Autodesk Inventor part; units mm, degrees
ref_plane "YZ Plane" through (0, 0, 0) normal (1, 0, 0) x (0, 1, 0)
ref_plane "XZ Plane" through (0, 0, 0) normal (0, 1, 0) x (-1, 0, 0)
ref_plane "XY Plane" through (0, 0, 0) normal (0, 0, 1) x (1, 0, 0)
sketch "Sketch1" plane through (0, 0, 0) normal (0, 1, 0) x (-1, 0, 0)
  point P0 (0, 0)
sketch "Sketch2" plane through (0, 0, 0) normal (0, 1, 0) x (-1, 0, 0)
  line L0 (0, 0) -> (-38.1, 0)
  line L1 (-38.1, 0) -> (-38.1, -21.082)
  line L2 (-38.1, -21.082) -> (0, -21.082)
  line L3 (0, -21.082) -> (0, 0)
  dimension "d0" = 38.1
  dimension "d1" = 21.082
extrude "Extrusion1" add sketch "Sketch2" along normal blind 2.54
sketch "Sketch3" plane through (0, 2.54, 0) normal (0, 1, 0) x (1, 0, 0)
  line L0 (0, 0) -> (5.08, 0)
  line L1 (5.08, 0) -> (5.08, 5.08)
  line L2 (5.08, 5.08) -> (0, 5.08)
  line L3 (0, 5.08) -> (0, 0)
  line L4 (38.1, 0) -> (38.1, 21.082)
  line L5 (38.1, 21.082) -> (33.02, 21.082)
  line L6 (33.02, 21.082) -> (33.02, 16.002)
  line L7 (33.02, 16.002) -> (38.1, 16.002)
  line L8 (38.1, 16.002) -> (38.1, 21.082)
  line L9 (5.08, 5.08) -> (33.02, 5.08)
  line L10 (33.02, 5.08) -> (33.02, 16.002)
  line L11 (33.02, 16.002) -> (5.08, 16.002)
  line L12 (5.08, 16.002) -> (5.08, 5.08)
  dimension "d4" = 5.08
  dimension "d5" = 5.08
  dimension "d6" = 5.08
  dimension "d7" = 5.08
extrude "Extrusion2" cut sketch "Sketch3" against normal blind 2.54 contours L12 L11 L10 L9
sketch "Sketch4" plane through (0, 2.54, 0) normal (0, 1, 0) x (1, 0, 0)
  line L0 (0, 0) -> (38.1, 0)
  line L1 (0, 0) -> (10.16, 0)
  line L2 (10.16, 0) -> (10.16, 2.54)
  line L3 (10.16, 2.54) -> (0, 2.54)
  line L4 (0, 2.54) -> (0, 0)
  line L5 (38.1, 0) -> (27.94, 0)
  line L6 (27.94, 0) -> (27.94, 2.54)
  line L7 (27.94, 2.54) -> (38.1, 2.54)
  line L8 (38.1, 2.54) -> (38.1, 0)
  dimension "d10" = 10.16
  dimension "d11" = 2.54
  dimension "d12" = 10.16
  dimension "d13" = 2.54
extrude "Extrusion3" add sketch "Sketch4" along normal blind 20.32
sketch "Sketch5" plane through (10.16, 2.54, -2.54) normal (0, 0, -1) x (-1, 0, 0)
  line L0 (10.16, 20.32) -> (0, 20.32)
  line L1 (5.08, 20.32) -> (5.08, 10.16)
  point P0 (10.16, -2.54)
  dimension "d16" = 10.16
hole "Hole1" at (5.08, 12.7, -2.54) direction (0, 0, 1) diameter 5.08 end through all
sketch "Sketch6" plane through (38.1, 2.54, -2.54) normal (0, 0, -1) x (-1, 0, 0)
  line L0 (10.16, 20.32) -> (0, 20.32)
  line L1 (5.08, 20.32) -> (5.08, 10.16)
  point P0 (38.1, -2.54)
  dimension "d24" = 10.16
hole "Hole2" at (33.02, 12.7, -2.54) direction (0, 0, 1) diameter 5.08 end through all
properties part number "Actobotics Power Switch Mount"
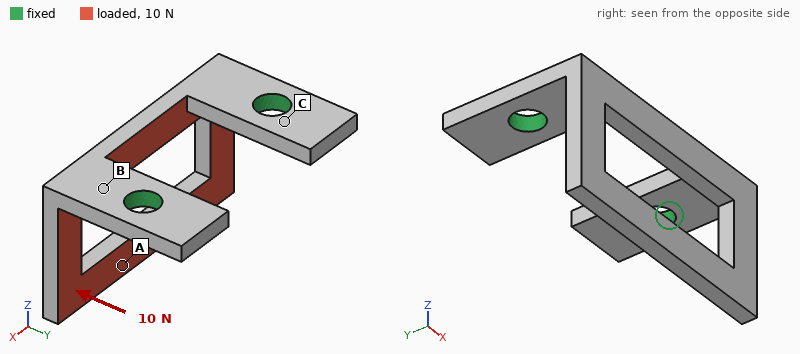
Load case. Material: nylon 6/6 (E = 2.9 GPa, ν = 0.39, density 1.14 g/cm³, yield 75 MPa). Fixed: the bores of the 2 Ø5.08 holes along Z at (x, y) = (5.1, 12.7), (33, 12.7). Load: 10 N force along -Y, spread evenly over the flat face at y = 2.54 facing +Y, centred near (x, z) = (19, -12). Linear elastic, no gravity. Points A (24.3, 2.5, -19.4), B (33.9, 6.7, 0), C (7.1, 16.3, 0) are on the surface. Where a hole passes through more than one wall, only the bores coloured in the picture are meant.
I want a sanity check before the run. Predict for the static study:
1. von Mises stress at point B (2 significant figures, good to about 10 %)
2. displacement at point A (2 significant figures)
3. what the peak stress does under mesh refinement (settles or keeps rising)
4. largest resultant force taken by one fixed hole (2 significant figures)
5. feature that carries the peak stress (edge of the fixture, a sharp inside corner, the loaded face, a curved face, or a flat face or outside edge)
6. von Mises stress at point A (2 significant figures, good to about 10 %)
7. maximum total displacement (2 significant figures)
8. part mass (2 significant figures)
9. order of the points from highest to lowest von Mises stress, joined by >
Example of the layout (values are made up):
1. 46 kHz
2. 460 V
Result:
1. 4.1 MPa
2. 0.44 mm
3. keeps rising
4. 5.0 N
5. a sharp inside corner
6. 1.4 MPa
7. 0.50 mm
8. 2.5 g
9. B > A > C
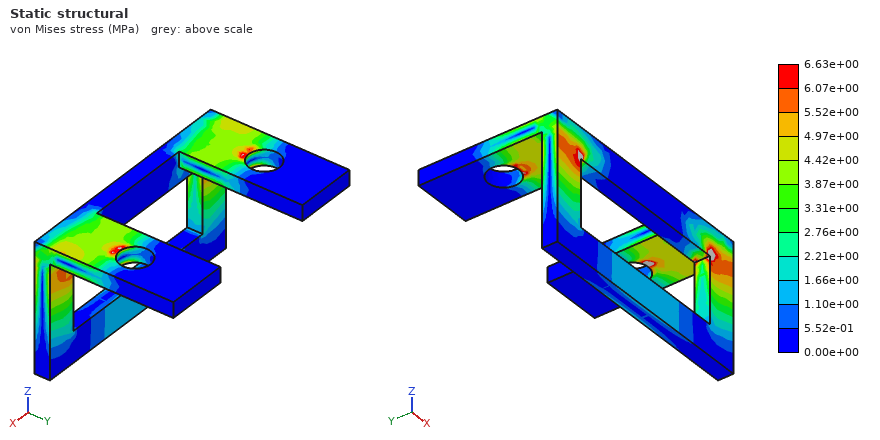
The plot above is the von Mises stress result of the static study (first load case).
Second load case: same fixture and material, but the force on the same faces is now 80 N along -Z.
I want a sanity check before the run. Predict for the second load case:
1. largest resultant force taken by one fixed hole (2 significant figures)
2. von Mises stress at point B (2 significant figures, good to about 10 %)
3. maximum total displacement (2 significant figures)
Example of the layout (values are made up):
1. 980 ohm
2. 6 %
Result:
1. 40 N
2. 14 MPa
3. 0.48 mm
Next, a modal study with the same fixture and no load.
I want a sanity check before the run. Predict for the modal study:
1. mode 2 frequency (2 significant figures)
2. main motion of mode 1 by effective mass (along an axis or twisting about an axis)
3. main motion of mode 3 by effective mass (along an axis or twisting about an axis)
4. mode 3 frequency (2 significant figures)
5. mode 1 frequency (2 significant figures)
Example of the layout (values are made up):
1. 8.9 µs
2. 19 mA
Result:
1. 1400 Hz
2. along Y
3. along X
4. 2100 Hz
5. 720 Hz
